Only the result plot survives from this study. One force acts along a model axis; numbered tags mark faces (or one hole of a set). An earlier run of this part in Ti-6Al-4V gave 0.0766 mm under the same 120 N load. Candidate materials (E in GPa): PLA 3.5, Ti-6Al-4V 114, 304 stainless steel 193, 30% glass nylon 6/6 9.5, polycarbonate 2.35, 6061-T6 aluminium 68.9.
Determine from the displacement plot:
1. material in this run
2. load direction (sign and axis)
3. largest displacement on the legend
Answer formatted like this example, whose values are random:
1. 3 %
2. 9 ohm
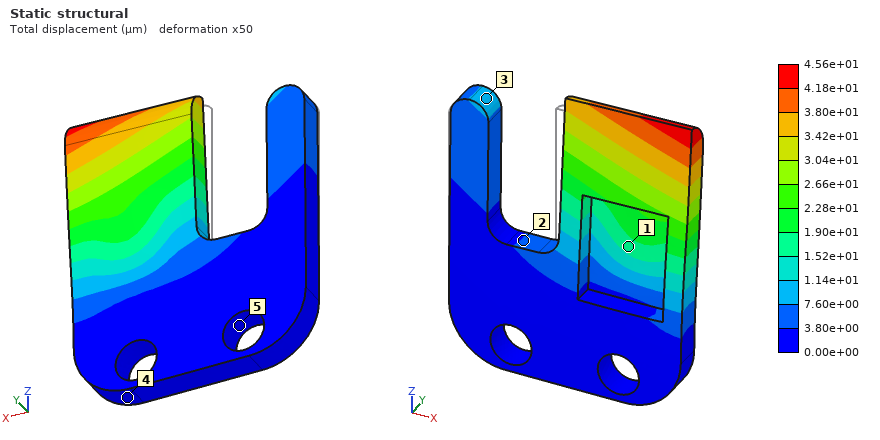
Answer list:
1. 304 stainless steel
2. +Y
3. 4.56e+01 µm
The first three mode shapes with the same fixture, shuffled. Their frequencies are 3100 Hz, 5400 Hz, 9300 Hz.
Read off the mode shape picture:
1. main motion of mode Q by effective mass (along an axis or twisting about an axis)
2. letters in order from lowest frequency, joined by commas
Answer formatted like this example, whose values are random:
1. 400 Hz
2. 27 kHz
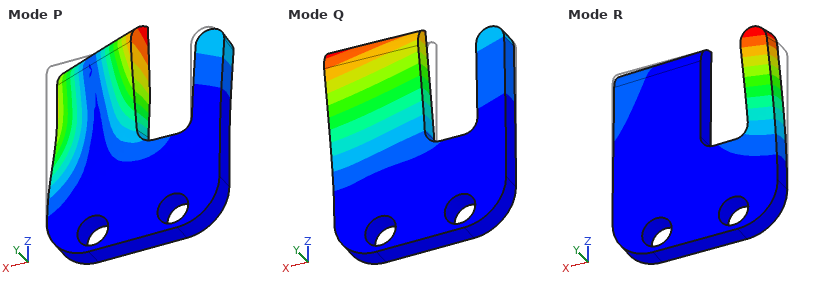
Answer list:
1. along Y
2. Q, R, P
